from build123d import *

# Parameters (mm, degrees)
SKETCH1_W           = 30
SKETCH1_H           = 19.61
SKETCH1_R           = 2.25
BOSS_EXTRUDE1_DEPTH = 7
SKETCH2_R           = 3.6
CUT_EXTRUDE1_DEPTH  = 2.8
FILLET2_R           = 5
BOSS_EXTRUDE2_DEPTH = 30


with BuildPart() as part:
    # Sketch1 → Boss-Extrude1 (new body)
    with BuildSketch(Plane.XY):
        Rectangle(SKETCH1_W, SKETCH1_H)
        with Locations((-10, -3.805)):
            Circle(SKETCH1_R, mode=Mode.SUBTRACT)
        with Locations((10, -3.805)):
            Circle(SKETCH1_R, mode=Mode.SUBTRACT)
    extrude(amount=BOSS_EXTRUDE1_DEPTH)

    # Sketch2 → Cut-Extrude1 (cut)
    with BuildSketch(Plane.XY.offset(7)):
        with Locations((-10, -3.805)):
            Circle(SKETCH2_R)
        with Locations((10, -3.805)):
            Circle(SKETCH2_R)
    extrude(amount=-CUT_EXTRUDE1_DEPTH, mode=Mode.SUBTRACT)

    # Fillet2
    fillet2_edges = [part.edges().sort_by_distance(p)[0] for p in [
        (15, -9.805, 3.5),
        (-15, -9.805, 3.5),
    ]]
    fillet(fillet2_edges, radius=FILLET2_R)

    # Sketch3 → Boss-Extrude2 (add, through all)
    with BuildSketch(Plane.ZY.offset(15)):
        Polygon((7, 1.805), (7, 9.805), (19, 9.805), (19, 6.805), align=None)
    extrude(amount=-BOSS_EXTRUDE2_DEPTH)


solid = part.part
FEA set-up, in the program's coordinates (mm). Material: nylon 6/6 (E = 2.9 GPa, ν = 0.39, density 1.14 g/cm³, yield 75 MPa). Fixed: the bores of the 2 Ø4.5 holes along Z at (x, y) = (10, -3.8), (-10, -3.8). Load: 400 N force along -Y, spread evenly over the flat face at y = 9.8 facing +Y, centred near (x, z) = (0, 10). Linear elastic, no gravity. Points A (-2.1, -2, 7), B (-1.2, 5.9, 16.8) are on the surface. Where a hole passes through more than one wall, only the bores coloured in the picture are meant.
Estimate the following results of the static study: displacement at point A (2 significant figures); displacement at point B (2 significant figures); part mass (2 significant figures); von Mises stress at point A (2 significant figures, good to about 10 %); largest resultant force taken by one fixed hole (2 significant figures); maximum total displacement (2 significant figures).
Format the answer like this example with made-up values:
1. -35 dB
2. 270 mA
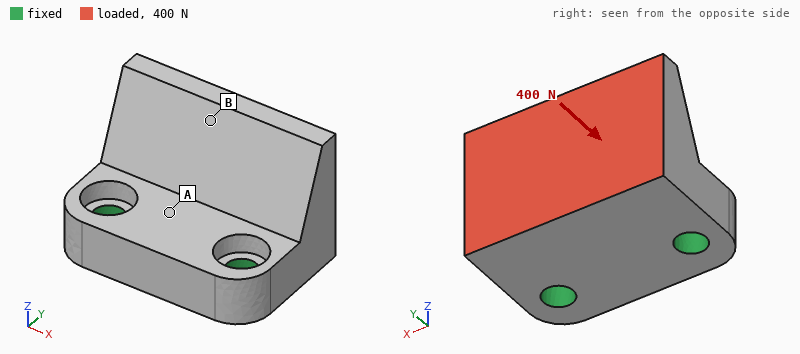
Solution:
1. 0.059 mm
2. 0.28 mm
3. 6.5 g
4. 8.0 MPa
5. 200 N
6. 0.36 mm
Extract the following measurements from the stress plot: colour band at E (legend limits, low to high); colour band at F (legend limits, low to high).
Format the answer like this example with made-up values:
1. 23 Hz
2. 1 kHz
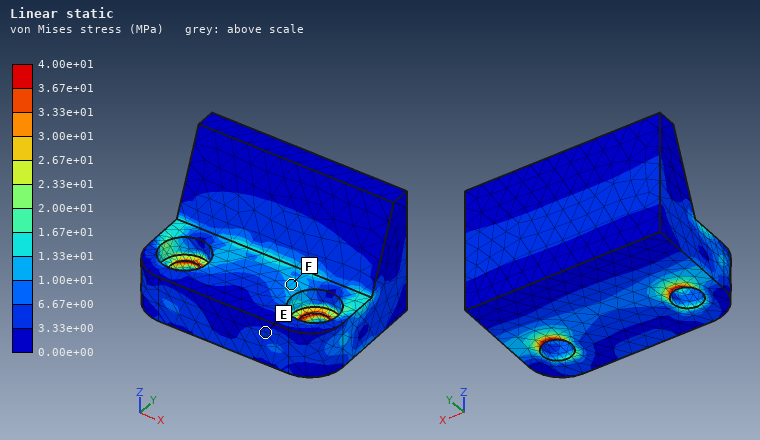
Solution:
1. 3.33e+00 to 6.67e+00 MPa
2. 1.00e+01 to 1.33e+01 MPa
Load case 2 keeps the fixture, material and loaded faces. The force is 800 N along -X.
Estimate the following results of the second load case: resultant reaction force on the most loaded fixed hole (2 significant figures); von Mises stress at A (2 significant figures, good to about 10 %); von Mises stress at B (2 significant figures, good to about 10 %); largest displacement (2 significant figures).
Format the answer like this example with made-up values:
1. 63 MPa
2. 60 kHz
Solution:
1. 680 N
2. 7.8 MPa
3. 3.3 MPa
4. 0.16 mm
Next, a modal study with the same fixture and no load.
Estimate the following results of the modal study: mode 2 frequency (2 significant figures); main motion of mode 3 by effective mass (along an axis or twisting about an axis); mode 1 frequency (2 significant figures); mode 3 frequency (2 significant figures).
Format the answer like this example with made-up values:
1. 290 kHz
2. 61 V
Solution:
1. 5700 Hz
2. along X
3. 2900 Hz
4. 8400 Hz
